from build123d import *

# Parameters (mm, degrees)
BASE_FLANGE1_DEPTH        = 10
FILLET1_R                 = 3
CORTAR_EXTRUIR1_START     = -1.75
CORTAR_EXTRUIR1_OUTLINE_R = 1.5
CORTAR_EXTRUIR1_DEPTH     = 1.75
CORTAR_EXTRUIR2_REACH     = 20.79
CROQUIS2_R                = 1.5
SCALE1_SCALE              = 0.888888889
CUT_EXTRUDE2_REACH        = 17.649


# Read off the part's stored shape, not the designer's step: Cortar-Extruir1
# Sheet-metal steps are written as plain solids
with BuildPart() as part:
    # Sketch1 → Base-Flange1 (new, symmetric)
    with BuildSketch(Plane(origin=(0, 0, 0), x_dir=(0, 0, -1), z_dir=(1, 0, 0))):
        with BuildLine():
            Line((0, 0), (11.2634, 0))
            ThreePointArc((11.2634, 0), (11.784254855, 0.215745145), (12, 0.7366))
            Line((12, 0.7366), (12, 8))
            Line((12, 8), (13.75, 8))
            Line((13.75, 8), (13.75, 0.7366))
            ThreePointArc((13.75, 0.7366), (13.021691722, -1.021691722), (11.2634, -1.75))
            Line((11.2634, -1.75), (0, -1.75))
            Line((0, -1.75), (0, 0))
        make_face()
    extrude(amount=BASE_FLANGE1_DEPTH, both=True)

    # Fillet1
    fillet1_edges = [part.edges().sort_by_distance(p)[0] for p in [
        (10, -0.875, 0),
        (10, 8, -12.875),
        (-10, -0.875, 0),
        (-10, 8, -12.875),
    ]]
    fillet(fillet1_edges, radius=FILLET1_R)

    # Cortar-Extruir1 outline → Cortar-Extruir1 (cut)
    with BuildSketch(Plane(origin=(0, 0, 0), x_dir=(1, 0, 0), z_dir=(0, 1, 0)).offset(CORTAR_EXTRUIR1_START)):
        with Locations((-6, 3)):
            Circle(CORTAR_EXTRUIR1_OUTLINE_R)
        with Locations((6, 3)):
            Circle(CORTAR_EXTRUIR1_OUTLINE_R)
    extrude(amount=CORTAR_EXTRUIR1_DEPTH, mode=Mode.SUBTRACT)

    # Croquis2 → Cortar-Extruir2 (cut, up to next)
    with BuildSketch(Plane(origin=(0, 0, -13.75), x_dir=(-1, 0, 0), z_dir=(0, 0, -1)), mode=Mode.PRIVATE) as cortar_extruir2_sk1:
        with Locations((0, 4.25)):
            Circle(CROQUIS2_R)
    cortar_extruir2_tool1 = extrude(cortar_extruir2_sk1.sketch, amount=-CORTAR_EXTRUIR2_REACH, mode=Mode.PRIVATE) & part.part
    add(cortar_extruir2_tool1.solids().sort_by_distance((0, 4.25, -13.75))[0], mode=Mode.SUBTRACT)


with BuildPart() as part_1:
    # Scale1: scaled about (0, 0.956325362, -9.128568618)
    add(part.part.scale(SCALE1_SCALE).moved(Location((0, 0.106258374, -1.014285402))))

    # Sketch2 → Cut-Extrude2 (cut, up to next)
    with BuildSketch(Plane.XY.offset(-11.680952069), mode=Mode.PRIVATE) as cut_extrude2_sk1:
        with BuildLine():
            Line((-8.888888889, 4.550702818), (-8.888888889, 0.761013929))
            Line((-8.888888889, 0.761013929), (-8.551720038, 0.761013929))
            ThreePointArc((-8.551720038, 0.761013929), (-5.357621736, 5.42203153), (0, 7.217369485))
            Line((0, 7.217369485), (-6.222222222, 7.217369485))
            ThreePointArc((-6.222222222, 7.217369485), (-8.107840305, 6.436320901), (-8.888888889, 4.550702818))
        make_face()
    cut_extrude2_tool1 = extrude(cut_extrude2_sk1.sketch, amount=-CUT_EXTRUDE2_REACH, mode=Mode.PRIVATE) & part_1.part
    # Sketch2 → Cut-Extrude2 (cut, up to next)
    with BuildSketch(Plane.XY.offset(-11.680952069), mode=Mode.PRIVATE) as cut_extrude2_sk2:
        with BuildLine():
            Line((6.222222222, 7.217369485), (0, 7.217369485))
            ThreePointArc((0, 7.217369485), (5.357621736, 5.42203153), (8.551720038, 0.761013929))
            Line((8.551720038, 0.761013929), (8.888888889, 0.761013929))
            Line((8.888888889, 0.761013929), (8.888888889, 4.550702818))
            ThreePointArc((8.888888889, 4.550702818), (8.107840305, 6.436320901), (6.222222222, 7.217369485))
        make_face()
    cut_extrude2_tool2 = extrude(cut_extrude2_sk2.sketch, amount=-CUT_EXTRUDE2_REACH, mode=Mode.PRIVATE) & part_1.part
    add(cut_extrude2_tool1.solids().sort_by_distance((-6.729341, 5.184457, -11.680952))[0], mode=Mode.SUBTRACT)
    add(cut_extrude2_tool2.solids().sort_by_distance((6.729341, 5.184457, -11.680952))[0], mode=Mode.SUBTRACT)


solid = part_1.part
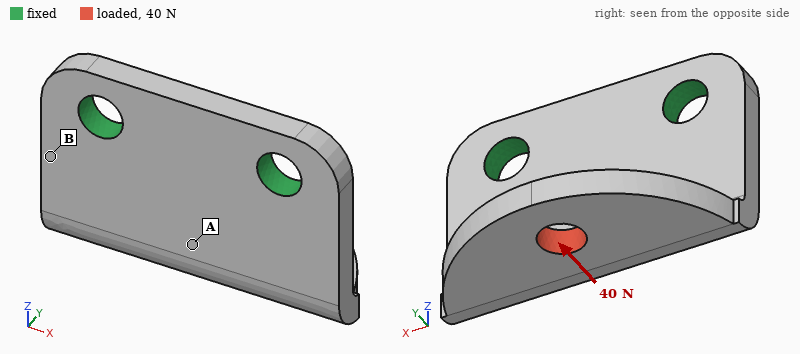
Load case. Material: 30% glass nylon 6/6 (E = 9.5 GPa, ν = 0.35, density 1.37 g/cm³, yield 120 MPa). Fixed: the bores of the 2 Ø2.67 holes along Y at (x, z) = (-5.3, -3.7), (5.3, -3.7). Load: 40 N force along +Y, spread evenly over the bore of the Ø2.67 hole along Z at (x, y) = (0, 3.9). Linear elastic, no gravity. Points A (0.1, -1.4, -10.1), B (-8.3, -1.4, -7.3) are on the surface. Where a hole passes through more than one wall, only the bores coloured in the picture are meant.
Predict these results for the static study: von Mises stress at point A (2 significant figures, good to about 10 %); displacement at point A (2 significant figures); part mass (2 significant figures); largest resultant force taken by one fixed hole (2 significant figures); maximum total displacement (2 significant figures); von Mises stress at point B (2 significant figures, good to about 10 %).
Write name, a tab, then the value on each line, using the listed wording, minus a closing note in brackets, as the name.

von Mises stress at point A	13 MPa
displacement at point A	0.084 mm
part mass	0.60 g
largest resultant force taken by one fixed hole	20 N
maximum total displacement	0.25 mm
von Mises stress at point B	30 MPa
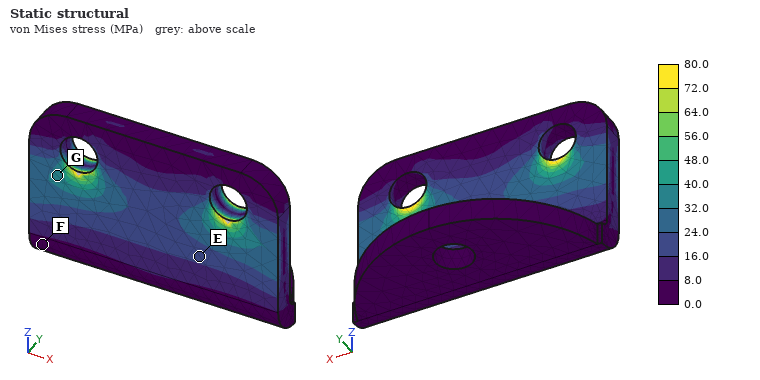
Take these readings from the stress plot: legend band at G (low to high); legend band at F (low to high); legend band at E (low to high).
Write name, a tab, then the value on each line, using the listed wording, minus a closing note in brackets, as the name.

legend band at G	32.0 to 40.0 MPa
legend band at F	0.0 to 8.0 MPa
legend band at E	16.0 to 24.0 MPa
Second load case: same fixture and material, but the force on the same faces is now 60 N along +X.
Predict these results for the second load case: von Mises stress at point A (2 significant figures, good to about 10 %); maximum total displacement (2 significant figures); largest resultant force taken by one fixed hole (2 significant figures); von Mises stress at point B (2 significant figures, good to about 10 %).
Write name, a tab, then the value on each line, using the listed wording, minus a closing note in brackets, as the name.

von Mises stress at point A	11 MPa
maximum total displacement	0.11 mm
largest resultant force taken by one fixed hole	54 N
von Mises stress at point B	19 MPa
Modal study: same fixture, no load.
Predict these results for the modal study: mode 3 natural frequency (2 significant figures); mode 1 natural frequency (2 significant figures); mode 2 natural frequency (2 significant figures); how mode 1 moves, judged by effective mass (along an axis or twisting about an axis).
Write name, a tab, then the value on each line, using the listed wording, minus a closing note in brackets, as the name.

mode 3 natural frequency	12 kHz
mode 1 natural frequency	4400 Hz
mode 2 natural frequency	7900 Hz
how mode 1 moves, judged by effective mass	along Y
